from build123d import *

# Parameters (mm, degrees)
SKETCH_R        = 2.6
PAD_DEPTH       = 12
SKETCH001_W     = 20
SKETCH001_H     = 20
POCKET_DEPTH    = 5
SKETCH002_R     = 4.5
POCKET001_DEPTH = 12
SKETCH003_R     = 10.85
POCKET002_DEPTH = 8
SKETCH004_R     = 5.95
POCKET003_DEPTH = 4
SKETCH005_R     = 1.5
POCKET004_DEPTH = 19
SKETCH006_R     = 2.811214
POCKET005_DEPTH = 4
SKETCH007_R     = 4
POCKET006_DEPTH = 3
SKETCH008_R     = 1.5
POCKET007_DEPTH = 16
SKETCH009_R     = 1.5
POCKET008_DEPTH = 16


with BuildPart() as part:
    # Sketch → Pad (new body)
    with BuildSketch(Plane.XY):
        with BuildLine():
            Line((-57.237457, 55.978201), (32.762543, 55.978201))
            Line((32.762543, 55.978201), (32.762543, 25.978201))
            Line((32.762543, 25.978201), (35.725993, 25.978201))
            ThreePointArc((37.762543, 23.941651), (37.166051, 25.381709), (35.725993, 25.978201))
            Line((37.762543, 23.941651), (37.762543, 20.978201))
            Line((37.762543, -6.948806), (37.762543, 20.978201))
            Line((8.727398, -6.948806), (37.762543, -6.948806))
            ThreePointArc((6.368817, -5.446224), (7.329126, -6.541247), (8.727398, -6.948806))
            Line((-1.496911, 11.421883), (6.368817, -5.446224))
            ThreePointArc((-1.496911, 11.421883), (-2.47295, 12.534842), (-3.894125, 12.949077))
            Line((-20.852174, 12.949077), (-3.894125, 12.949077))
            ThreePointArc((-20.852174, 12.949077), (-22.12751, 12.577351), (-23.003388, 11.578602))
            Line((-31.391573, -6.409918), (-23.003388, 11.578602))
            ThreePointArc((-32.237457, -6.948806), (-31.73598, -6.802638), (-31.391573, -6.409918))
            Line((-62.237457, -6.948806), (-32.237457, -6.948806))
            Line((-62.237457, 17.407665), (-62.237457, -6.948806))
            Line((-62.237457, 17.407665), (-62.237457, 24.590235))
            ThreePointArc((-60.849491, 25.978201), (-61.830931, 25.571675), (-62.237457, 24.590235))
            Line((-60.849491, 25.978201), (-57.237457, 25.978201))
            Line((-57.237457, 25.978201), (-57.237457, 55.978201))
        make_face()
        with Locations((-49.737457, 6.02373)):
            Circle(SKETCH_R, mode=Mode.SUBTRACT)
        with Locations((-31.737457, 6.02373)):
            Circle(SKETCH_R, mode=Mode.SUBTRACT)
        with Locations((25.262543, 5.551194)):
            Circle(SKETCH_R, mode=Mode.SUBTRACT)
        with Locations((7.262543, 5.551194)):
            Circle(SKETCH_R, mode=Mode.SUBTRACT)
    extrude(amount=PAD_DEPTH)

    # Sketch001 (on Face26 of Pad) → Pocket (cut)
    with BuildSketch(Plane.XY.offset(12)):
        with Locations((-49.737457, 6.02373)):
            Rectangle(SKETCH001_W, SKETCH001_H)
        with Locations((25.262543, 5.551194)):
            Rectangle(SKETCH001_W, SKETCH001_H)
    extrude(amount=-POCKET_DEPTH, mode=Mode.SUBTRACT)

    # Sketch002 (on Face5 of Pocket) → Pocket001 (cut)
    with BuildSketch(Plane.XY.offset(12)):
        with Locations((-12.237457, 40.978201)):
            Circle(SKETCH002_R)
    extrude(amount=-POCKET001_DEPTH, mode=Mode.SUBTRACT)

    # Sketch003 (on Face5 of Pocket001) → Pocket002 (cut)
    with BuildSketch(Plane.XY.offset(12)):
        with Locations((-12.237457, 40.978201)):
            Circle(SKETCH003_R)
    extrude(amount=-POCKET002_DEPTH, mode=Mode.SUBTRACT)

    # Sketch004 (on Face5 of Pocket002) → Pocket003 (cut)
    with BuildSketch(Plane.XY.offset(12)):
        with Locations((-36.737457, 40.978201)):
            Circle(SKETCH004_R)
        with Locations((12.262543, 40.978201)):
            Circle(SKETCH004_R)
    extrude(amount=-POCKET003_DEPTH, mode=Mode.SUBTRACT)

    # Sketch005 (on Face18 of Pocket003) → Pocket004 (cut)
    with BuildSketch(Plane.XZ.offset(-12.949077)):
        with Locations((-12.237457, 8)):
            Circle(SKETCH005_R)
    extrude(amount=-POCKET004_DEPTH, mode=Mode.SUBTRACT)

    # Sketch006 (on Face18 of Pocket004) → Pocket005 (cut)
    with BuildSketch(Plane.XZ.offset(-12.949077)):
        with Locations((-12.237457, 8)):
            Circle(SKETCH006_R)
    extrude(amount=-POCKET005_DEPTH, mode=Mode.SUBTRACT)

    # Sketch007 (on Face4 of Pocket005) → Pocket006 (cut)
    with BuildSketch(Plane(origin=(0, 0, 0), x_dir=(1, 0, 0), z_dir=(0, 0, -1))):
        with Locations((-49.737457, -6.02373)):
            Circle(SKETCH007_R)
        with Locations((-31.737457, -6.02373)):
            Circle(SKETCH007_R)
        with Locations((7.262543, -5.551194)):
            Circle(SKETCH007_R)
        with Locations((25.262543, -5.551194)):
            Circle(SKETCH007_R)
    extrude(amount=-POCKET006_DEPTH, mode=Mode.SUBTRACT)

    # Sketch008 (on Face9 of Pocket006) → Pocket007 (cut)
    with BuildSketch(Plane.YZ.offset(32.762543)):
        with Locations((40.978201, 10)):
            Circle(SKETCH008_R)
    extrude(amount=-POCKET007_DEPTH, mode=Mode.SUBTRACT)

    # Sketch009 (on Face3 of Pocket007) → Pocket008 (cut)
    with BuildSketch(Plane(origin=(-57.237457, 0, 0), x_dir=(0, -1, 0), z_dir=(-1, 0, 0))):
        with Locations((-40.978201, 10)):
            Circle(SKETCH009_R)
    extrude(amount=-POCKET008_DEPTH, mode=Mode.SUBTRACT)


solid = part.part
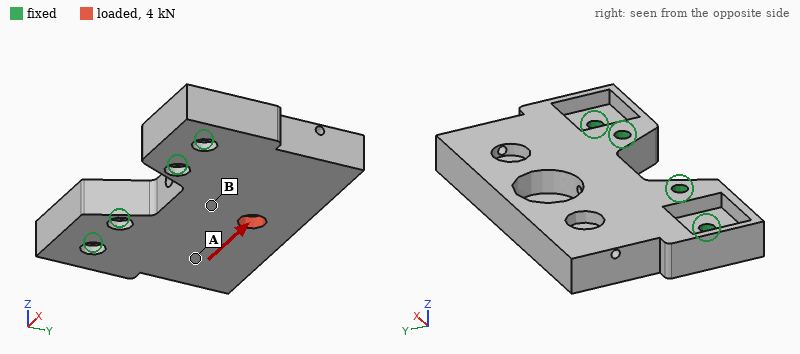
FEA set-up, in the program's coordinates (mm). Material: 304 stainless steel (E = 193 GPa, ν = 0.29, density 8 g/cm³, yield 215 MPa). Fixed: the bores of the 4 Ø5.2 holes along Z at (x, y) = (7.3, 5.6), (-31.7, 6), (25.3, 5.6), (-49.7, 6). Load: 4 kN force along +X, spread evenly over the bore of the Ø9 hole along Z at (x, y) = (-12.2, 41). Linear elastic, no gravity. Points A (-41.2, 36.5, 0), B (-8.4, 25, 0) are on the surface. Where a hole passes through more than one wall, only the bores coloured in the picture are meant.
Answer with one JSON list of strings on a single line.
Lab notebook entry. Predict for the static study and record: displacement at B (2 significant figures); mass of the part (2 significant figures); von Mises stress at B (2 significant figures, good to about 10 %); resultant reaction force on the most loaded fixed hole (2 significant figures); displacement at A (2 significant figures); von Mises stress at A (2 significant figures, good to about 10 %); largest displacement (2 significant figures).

["2.5 µm", "440 g", "19 MPa", "1.7 kN", "4.4 µm", "8.5 MPa", "8.0 µm"]
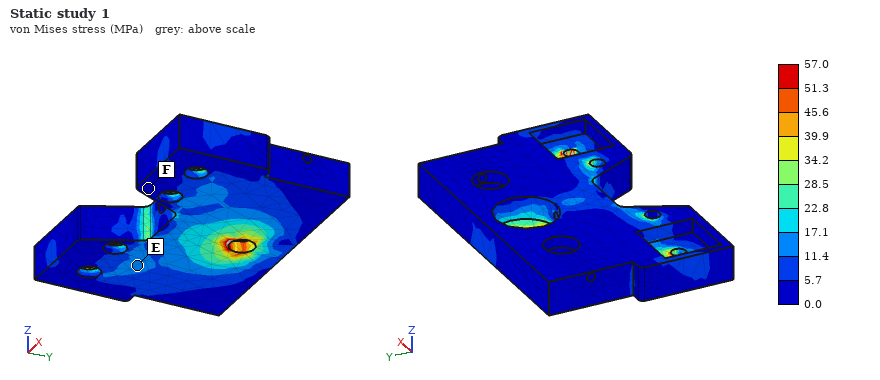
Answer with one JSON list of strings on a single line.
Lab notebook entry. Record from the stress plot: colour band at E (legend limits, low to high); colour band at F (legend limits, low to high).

["11.4 to 17.1 MPa", "0.0 to 5.7 MPa"]
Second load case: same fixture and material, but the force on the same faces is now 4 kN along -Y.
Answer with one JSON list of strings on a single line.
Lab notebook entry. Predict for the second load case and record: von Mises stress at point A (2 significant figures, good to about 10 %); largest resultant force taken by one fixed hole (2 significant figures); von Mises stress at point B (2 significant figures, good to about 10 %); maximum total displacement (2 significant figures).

["7.4 MPa", "1.4 kN", "18 MPa", "16 µm"]
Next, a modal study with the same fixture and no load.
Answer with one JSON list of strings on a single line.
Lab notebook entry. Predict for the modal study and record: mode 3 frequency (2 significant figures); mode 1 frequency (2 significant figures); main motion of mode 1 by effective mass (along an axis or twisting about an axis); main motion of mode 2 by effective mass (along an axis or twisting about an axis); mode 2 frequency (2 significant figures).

["9000 Hz", "2600 Hz", "along Z", "twisting about Y", "4200 Hz"]
